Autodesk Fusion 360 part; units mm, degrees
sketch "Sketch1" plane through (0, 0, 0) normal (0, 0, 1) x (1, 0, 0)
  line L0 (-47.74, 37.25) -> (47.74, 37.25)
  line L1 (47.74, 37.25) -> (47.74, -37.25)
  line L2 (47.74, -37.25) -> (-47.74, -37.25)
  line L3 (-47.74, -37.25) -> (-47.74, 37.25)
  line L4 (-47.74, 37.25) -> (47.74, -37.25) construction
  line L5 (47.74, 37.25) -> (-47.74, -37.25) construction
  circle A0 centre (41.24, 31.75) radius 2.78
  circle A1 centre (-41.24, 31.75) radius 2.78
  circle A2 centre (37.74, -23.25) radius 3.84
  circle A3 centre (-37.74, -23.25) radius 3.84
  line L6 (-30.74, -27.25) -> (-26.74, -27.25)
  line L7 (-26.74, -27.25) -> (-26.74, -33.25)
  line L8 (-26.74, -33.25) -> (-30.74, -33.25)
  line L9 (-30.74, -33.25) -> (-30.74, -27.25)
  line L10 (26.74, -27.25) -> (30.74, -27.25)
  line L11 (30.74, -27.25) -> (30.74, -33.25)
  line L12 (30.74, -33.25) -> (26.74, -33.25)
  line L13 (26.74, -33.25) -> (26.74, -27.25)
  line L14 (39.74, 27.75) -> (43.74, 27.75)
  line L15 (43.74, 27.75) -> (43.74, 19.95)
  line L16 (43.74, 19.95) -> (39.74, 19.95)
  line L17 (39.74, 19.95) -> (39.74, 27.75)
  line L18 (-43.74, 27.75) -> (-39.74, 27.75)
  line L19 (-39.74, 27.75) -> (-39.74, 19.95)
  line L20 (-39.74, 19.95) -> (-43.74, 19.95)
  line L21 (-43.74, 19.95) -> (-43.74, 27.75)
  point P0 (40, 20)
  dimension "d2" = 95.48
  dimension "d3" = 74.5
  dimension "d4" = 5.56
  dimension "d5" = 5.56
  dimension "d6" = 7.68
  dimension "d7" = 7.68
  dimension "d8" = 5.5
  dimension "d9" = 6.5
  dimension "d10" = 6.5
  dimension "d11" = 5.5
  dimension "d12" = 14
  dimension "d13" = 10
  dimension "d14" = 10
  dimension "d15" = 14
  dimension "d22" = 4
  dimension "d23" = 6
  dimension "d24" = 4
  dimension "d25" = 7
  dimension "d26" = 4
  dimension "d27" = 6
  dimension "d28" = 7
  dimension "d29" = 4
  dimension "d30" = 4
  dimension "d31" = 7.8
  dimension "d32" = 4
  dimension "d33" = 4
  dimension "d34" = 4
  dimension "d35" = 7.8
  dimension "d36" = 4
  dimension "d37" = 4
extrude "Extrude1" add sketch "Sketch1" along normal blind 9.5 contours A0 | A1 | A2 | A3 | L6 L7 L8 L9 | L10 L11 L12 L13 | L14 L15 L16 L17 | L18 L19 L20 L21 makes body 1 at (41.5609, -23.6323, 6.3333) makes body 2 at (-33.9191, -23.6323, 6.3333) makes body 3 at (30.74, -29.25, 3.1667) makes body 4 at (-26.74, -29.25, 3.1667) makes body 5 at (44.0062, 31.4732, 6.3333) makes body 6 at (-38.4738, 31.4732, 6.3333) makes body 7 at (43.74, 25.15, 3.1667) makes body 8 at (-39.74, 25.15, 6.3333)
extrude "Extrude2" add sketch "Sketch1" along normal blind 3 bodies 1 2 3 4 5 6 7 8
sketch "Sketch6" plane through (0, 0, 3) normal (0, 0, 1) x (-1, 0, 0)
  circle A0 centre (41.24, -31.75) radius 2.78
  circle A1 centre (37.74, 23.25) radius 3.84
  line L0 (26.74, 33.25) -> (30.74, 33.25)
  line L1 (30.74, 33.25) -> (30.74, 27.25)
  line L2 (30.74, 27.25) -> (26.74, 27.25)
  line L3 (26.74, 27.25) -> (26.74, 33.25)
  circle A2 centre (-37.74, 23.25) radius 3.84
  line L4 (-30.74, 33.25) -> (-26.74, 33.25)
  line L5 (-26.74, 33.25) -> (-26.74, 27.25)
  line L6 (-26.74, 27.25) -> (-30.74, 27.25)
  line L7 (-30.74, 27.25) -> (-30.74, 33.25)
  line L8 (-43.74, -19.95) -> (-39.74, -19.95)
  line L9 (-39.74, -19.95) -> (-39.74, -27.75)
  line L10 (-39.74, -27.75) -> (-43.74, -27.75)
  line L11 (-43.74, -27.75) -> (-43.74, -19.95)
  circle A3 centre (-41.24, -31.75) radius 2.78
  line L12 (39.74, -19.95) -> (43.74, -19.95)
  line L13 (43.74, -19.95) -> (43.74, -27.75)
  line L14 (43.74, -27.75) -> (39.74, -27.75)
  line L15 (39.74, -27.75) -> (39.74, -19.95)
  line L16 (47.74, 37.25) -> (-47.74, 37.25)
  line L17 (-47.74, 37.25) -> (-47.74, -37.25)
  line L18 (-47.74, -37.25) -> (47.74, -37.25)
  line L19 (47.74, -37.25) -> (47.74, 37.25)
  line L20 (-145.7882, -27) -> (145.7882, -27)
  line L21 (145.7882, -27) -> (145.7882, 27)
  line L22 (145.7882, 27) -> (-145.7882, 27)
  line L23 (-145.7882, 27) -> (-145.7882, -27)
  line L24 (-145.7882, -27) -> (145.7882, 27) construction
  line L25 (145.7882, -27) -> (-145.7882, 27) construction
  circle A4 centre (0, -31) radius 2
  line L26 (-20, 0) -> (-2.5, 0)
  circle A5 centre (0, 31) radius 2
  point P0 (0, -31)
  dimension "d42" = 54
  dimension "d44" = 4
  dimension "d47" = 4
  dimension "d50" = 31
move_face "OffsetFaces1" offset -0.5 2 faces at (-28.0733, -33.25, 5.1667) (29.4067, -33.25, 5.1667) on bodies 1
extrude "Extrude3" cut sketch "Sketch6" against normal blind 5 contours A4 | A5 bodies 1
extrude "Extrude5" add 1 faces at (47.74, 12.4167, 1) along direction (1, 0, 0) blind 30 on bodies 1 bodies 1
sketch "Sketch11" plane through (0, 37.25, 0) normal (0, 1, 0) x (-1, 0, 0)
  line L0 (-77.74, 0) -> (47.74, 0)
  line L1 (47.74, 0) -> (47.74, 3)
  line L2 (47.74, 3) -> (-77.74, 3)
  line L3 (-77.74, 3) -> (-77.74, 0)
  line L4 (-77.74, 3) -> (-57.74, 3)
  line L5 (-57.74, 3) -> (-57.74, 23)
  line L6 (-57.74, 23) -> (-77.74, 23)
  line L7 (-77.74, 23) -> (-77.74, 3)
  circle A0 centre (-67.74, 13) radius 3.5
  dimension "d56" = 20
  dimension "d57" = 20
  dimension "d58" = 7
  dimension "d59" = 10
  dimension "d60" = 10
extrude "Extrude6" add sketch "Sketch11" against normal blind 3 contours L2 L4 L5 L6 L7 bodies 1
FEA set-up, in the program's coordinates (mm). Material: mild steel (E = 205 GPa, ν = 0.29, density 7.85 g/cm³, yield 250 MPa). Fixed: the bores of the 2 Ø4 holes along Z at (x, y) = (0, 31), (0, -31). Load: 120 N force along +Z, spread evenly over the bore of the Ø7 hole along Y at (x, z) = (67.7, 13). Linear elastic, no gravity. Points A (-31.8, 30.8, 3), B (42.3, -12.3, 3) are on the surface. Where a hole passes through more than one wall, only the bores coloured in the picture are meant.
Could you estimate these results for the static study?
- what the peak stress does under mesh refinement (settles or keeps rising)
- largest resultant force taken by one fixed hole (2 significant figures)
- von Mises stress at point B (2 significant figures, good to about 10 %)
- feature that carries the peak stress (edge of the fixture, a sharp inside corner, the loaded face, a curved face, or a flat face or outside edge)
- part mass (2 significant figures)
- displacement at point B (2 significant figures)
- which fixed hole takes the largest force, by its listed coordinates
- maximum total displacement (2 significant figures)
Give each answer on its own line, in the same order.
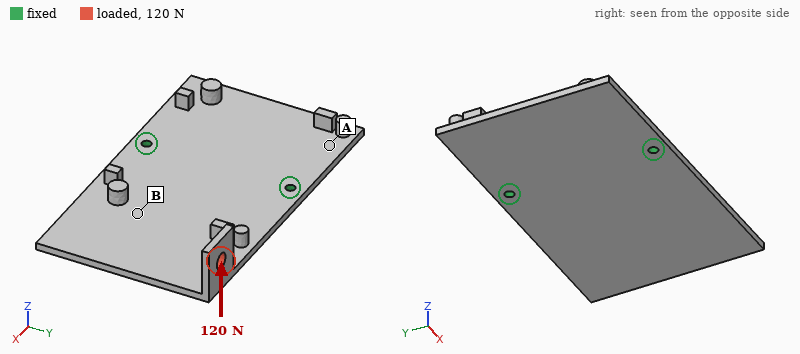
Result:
keeps rising
130 N
32 MPa
edge of the fixture
240 g
0.19 mm
(0, 31)
0.71 mm
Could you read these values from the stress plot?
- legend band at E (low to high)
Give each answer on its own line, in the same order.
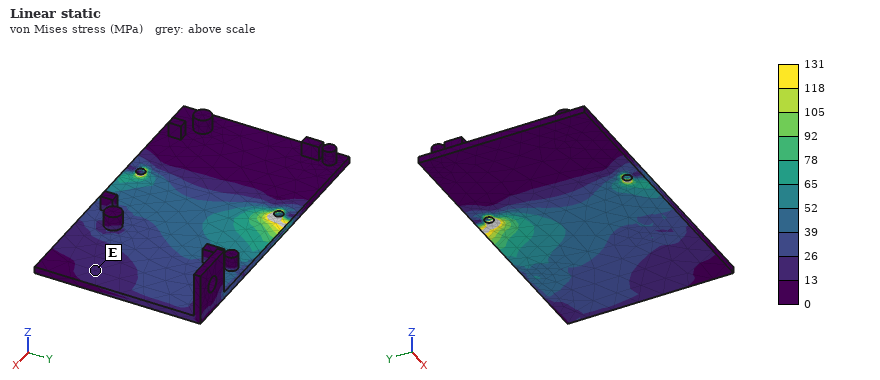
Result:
13 to 26 MPa
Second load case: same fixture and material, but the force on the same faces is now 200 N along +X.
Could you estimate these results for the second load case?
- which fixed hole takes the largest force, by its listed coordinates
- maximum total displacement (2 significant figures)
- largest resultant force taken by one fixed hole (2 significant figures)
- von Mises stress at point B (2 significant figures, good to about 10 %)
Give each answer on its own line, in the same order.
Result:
(0, 31)
0.31 mm
210 N
16 MPa
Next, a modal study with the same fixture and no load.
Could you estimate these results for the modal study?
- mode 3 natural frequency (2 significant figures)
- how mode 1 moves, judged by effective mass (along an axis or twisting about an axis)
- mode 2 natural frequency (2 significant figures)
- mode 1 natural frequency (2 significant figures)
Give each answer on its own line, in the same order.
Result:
900 Hz
along Z
870 Hz
330 Hz
